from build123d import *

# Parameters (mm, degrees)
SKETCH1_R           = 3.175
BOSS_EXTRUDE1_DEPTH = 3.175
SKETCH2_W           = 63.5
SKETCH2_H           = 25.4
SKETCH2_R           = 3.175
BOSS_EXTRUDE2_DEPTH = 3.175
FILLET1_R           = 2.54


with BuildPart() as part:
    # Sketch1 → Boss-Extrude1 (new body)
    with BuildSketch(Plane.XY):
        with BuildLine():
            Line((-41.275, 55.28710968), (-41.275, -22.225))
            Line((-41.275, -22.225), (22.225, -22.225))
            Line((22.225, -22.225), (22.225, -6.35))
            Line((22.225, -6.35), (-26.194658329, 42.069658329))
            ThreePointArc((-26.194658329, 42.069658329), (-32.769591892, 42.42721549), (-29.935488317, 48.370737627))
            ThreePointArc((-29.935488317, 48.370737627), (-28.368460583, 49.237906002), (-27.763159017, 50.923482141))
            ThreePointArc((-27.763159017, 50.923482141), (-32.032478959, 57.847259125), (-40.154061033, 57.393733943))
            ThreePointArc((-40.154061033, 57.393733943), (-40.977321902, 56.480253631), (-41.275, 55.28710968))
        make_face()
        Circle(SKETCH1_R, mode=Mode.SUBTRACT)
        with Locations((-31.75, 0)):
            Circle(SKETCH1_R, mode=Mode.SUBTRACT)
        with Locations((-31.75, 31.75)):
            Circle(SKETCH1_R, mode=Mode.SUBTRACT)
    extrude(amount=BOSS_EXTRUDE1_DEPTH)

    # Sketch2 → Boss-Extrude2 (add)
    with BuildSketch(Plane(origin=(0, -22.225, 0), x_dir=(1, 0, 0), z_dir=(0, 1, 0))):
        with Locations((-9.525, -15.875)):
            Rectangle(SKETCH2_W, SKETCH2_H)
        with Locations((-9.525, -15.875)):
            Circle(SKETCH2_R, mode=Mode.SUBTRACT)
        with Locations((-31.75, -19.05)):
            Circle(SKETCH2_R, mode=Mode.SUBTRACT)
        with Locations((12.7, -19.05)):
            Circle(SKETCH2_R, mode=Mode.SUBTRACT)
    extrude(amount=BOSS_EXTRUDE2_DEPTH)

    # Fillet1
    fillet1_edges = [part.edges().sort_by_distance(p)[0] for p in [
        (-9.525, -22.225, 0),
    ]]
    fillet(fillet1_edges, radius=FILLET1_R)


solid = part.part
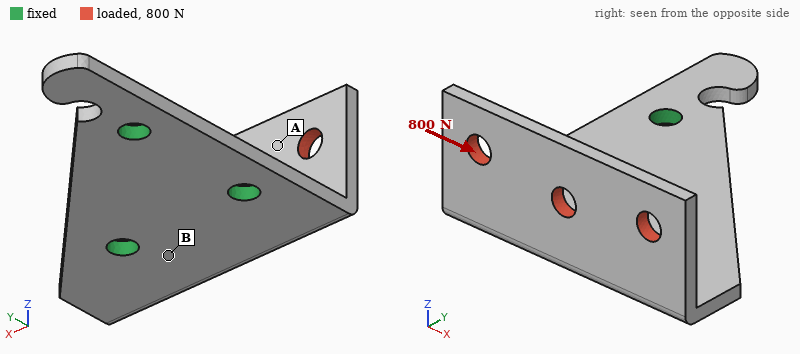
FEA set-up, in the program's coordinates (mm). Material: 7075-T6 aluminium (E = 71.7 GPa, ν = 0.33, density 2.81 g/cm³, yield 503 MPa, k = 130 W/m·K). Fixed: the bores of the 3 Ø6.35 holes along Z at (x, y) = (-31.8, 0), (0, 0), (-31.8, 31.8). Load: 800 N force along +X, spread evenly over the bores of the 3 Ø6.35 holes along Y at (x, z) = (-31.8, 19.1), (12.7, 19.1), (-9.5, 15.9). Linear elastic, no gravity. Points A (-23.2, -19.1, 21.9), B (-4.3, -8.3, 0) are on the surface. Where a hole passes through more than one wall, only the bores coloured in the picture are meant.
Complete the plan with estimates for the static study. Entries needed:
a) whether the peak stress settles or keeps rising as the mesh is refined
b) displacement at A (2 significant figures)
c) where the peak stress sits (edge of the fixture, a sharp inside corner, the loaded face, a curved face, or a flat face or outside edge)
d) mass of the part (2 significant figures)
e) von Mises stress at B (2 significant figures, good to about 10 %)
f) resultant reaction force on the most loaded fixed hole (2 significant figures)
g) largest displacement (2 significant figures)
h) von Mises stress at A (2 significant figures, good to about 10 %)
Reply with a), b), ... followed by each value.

a) keeps rising
b) 0.12 mm
c) edge of the fixture
d) 40 g
e) 44 MPa
f) 690 N
g) 0.25 mm
h) 17 MPa
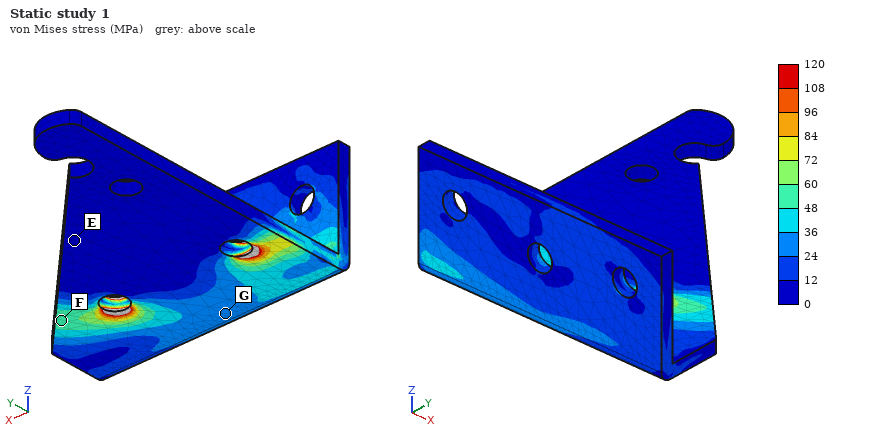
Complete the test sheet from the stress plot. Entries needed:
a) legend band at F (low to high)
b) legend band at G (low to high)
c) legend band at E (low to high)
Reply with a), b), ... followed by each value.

a) 48 to 60 MPa
b) 24 to 36 MPa
c) 0 to 12 MPa
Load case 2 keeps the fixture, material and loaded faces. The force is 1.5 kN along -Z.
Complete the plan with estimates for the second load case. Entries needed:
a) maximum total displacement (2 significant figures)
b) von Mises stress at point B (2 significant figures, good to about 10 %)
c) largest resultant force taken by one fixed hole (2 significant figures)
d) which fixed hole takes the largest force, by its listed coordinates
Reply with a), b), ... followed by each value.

a) 0.85 mm
b) 210 MPa
c) 1.0 kN
d) (0, 0)
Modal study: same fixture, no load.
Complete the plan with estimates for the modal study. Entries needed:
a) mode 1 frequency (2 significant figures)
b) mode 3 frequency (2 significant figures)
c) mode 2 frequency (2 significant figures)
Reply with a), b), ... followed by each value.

a) 1600 Hz
b) 4100 Hz
c) 2500 Hz
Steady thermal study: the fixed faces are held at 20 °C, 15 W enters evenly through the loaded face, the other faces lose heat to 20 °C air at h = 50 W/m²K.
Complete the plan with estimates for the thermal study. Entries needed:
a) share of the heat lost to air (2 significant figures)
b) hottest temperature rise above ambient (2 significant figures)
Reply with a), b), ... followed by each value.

a) 24 %
b) 21 K
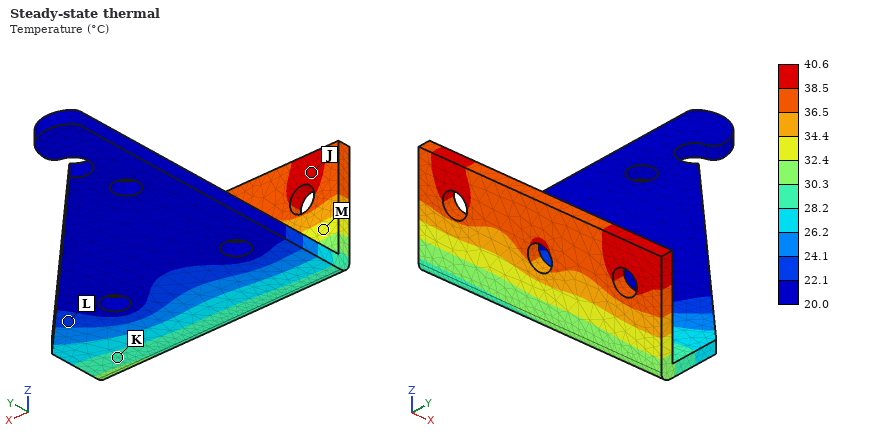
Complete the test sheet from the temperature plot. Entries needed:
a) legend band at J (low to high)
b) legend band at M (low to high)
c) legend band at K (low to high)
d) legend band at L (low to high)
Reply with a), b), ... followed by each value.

a) 38.5 to 40.6 °C
b) 32.4 to 34.4 °C
c) 28.2 to 30.3 °C
d) 22.1 to 24.1 °C
